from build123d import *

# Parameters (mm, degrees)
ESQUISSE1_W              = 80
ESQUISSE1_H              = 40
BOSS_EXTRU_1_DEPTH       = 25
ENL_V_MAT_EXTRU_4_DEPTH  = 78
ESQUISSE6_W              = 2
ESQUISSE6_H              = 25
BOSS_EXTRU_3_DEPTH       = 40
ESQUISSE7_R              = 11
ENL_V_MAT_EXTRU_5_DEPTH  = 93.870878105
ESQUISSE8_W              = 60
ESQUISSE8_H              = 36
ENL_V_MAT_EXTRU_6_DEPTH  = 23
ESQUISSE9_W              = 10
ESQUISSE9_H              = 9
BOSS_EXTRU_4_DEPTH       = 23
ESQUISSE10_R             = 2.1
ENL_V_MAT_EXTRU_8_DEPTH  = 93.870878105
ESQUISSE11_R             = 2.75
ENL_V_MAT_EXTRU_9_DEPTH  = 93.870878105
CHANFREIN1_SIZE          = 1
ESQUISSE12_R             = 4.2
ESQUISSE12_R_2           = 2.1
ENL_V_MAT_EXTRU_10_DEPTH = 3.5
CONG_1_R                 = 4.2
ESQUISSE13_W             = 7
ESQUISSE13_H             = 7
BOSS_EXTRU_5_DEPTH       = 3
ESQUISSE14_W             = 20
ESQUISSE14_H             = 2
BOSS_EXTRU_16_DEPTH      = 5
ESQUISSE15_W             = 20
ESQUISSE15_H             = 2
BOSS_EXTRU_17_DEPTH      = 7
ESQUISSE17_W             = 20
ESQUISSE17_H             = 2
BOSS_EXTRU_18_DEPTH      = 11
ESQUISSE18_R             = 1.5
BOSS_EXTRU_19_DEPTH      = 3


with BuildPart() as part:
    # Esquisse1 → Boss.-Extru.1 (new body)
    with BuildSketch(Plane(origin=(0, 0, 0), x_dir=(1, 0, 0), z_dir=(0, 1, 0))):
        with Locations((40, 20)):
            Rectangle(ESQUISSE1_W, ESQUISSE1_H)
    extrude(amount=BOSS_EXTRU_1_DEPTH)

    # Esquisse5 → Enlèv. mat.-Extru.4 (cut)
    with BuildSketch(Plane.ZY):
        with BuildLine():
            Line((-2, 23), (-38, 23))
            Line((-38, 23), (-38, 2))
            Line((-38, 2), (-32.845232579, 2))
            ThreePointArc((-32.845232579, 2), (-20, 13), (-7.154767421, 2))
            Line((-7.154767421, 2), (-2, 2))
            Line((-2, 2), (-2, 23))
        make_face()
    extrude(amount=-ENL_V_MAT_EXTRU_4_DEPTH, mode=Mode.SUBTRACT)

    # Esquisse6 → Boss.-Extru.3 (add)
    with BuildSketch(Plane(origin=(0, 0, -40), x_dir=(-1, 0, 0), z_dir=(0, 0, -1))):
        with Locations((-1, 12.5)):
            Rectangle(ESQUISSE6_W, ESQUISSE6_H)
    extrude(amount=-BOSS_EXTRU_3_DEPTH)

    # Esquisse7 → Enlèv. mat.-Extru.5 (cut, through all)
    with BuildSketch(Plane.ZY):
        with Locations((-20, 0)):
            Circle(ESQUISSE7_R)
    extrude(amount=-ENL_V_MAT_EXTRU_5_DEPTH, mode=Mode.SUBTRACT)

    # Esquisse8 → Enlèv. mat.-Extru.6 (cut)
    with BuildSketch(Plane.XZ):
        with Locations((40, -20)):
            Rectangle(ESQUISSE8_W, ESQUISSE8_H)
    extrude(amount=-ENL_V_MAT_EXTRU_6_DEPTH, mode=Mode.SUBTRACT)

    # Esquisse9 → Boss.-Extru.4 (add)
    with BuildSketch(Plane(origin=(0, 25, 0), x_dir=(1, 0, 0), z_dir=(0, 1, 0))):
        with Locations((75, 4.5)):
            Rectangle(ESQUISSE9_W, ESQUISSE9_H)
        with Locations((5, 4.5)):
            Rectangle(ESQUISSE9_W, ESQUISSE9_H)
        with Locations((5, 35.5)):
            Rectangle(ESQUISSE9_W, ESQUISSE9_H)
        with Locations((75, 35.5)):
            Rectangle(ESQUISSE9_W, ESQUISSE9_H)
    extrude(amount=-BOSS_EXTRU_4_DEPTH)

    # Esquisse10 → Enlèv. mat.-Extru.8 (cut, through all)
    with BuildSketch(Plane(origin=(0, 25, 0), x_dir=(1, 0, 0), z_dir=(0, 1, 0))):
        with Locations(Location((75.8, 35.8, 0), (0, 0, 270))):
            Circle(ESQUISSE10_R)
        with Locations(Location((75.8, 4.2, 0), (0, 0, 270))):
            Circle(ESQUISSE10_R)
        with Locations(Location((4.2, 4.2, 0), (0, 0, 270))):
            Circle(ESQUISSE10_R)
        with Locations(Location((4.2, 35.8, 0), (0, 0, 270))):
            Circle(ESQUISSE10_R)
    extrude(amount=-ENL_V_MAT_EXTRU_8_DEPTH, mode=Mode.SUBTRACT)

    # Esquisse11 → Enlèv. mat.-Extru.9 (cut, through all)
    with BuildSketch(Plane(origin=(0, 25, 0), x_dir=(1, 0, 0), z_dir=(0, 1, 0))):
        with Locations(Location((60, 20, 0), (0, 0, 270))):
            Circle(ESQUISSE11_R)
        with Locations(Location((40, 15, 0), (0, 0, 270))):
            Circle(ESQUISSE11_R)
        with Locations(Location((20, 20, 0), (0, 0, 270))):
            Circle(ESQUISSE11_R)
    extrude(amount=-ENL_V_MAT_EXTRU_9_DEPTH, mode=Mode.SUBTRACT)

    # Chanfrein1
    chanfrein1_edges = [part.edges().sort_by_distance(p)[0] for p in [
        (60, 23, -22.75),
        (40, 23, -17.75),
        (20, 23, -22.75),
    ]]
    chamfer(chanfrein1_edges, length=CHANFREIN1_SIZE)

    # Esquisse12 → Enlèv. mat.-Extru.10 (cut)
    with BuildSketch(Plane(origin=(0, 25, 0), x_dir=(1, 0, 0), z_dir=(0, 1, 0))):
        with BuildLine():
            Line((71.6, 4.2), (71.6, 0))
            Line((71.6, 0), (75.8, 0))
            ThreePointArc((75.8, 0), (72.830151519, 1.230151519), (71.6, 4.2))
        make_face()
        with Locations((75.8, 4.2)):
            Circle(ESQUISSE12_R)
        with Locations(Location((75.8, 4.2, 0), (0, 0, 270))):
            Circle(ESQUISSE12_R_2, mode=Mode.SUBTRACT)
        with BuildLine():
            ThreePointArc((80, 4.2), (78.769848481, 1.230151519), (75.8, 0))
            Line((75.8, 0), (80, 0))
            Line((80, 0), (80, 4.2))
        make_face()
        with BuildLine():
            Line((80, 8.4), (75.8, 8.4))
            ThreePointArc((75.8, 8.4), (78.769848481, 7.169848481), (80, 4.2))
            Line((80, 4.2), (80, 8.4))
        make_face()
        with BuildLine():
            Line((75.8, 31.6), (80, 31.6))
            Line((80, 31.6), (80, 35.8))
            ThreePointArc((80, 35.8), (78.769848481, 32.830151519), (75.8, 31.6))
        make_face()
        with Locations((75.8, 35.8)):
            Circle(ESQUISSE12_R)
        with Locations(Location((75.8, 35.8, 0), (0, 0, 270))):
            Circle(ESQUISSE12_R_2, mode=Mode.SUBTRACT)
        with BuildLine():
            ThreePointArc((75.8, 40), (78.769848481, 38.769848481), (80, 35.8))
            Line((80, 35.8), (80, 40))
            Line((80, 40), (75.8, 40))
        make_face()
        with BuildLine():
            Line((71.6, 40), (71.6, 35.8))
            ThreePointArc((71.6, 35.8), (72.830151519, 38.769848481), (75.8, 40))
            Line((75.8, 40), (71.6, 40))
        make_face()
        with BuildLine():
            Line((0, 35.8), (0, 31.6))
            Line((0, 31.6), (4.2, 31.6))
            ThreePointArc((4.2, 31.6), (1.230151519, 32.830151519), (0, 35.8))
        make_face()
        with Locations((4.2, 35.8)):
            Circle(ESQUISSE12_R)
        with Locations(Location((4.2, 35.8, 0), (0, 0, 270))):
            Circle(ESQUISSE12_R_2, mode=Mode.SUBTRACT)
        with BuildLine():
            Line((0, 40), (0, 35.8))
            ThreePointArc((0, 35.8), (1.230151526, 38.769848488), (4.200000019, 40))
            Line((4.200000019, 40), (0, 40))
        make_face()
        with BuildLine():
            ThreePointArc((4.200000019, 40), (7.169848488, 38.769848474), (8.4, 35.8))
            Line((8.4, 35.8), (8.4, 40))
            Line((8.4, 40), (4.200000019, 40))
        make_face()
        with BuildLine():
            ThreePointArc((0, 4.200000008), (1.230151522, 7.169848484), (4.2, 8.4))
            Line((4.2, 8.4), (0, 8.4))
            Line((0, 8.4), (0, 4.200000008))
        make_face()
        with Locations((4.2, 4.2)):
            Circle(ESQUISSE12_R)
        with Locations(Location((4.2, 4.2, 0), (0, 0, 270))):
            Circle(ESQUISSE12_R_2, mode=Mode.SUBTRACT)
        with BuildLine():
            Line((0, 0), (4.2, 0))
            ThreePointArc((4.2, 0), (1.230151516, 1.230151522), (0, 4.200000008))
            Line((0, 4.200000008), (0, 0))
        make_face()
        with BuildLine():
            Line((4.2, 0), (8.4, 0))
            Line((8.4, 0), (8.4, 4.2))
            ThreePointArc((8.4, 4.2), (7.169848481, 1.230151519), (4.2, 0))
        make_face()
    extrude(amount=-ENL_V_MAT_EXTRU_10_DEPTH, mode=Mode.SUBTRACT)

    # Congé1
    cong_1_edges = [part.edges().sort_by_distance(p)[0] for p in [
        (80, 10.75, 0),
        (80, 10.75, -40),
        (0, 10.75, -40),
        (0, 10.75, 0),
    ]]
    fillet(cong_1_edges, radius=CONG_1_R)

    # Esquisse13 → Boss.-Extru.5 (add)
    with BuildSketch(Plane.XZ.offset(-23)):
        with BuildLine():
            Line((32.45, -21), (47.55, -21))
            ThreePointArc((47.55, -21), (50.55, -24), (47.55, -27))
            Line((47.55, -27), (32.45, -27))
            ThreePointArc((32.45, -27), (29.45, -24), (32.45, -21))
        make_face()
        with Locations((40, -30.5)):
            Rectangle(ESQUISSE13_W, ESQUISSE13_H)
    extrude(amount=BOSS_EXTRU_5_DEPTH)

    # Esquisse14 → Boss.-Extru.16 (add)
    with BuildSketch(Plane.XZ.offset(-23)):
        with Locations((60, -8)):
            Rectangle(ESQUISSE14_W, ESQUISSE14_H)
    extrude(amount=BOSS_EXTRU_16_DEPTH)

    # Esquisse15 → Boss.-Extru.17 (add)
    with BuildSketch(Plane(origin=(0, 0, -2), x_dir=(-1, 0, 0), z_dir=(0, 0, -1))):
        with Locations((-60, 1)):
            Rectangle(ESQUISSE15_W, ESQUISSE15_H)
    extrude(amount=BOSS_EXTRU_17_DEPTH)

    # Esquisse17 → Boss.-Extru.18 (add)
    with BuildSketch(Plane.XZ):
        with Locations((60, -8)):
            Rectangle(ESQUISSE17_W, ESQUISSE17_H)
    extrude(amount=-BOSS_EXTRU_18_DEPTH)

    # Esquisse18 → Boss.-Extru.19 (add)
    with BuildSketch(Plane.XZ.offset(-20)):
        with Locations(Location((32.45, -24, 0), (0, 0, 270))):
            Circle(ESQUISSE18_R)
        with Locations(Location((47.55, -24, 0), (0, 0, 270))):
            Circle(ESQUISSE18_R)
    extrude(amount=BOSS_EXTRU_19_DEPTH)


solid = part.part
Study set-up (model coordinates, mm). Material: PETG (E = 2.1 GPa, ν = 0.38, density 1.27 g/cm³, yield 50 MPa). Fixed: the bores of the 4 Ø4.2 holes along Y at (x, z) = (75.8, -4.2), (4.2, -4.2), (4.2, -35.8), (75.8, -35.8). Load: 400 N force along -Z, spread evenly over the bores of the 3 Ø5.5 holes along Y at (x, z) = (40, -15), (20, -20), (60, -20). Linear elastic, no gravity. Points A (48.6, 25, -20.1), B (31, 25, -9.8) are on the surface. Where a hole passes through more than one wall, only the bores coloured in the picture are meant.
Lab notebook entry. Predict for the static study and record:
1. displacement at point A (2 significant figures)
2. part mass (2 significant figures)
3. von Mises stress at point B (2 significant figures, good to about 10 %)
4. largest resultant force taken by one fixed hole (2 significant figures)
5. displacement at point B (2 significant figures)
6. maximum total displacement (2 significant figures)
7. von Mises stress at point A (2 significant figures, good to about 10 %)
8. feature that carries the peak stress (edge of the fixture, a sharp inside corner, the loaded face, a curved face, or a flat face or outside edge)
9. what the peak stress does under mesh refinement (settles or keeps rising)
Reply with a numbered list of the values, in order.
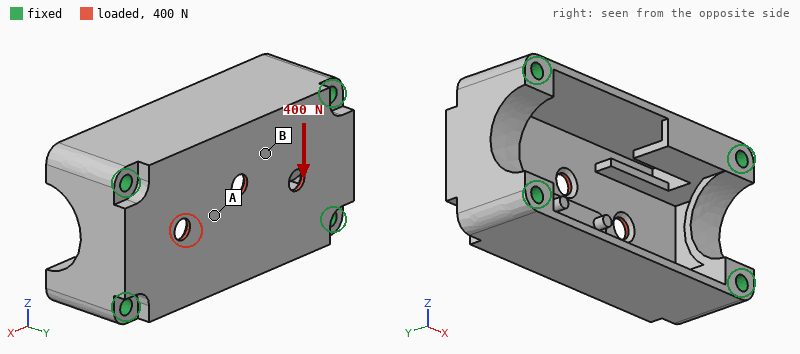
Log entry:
1. 0.11 mm
2. 27 g
3. 1.5 MPa
4. 120 N
5. 0.12 mm
6. 0.14 mm
7. 3.0 MPa
8. a sharp inside corner
9. keeps rising
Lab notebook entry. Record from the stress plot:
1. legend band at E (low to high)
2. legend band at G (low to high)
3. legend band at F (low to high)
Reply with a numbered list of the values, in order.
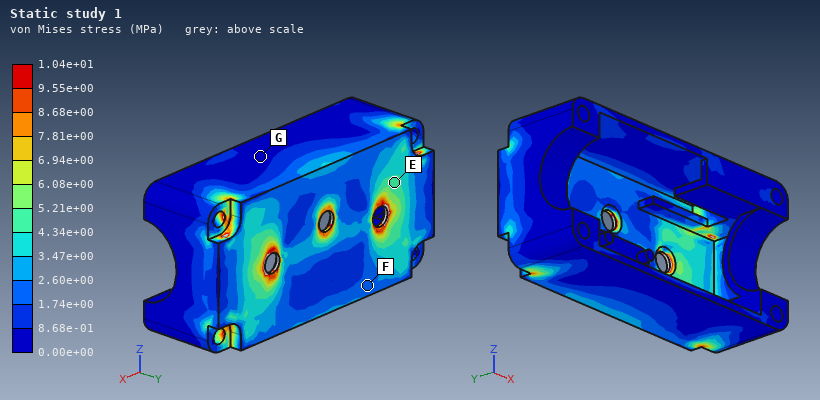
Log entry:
1. 4.34e+00 to 5.21e+00 MPa
2. 0.00e+00 to 8.68e-01 MPa
3. 1.74e+00 to 2.60e+00 MPa
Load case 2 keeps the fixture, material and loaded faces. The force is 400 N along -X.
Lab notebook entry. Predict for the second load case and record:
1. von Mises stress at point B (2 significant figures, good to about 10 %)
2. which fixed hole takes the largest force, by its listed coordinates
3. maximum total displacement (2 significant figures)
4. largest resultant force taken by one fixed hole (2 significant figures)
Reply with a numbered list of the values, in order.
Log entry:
1. 2.5 MPa
2. (75.8, -4.2)
3. 60 µm
4. 120 N
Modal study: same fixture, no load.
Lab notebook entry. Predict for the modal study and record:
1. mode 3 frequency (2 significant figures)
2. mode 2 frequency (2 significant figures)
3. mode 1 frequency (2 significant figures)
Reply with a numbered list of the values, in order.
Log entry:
1. 1800 Hz
2. 1400 Hz
3. 1100 Hz
